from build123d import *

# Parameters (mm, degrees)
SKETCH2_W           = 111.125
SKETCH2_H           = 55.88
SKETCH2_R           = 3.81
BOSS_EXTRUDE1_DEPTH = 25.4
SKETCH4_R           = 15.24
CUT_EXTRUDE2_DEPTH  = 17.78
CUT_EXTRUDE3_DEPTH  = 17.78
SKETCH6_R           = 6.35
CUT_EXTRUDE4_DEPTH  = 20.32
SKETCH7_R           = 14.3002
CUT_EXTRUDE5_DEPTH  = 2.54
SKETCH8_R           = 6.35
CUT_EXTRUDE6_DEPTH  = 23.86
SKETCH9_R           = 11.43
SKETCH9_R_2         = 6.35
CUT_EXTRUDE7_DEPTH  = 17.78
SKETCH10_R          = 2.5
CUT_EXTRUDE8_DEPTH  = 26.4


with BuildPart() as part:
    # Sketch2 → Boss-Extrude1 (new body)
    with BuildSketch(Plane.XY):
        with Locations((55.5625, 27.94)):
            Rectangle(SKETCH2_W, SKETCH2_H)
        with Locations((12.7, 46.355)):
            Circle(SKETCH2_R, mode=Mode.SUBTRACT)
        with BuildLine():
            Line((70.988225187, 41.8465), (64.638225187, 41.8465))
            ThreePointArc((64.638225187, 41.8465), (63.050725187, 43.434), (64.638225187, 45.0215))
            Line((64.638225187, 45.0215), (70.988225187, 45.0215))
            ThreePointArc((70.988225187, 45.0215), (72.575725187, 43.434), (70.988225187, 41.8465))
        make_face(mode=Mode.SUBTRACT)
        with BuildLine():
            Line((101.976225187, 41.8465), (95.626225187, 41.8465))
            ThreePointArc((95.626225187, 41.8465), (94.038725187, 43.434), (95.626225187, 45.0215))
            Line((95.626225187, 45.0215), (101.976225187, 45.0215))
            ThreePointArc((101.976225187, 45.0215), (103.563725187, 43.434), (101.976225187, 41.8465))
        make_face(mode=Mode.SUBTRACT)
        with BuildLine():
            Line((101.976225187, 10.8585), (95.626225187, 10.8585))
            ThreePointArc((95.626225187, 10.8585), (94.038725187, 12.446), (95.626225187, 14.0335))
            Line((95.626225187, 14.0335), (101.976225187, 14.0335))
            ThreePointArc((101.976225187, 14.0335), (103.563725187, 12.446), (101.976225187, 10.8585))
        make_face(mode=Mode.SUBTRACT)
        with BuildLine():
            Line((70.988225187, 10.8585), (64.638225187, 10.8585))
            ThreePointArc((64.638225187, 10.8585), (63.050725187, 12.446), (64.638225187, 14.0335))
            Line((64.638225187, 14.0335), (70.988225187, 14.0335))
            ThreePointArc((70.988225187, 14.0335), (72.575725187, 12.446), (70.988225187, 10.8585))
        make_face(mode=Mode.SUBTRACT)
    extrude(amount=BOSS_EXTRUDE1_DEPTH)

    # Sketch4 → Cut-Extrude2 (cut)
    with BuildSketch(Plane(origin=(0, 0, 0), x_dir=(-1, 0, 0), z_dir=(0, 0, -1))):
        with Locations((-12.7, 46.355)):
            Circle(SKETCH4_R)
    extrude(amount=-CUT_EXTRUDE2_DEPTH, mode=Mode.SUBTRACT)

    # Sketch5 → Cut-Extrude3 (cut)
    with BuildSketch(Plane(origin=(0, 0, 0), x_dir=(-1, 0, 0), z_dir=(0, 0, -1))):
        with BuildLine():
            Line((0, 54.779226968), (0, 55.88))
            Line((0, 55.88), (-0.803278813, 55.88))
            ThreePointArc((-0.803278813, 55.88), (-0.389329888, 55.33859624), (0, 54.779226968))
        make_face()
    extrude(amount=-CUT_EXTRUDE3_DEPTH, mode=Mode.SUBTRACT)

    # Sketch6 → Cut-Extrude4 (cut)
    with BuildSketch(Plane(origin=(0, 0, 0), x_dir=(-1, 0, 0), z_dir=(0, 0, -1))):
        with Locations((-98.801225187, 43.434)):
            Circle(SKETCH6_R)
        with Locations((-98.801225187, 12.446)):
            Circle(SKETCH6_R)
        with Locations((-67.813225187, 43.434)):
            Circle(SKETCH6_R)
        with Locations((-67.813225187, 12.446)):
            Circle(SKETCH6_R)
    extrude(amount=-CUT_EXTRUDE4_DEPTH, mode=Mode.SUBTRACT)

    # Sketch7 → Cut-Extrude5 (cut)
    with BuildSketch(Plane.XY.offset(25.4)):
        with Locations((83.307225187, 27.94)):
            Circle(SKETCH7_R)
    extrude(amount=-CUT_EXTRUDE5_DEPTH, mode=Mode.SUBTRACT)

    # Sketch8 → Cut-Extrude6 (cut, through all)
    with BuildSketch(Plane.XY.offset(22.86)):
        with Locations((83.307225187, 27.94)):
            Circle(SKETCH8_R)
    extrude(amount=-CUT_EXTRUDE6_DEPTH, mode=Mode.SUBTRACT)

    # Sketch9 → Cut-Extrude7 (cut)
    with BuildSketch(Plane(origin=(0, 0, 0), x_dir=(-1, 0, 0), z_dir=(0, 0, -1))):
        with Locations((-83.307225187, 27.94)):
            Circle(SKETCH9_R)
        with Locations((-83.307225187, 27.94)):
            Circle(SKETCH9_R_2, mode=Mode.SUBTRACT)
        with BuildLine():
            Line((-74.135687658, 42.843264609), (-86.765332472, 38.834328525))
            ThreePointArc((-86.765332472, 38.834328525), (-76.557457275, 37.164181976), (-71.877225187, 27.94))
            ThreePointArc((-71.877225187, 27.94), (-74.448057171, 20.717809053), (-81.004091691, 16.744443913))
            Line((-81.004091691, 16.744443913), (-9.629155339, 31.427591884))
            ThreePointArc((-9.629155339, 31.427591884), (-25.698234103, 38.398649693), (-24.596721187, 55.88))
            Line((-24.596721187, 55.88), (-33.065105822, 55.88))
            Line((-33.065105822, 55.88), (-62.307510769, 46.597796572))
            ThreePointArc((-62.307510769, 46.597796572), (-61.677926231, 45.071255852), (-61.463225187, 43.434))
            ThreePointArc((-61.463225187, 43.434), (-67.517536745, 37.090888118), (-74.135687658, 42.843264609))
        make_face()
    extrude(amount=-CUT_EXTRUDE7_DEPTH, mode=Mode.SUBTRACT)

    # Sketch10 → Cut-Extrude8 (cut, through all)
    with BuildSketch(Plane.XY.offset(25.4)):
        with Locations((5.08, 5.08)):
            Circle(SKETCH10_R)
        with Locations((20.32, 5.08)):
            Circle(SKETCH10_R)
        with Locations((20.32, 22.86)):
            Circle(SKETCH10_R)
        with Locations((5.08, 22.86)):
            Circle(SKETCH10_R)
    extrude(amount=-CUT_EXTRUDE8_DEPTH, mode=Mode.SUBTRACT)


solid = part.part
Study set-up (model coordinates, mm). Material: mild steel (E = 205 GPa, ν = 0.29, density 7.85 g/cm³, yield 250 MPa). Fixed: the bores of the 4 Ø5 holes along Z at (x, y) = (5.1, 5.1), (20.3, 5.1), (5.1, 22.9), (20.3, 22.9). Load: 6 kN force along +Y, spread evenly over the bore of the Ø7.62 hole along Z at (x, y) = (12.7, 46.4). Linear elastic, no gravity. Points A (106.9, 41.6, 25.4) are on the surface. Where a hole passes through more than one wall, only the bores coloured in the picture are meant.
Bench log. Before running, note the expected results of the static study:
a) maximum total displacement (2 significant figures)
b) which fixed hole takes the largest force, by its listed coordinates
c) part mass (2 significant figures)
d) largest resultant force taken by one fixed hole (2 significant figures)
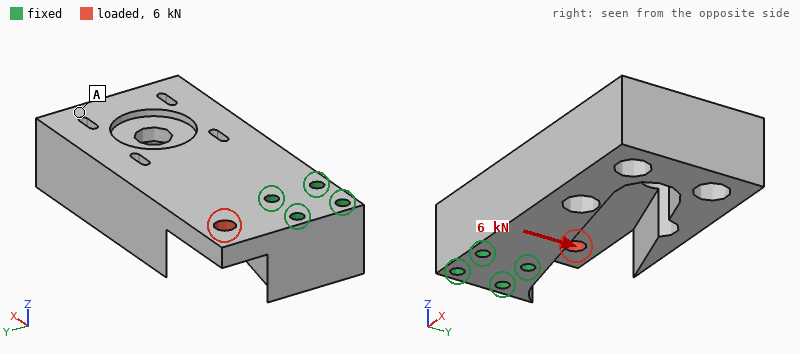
5.9 µm
(5.1, 22.9)
800 g
3.0 kN
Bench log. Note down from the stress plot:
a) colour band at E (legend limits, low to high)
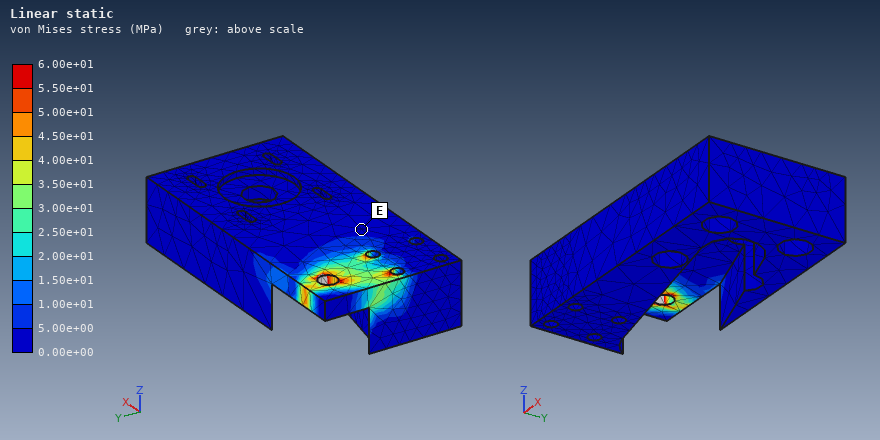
0.00e+00 to 5.00e+00 MPa
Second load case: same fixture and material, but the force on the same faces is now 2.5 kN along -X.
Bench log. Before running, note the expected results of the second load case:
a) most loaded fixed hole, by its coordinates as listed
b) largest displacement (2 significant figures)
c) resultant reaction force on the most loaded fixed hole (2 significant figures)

(20.3, 22.9)
7.5 µm
3.1 kN
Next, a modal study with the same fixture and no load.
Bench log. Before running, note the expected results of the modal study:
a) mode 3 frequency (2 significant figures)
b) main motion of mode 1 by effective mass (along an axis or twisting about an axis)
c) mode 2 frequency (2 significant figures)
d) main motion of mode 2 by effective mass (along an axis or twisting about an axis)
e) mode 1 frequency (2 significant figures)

3600 Hz
along Z
2700 Hz
along Y
1500 Hz
